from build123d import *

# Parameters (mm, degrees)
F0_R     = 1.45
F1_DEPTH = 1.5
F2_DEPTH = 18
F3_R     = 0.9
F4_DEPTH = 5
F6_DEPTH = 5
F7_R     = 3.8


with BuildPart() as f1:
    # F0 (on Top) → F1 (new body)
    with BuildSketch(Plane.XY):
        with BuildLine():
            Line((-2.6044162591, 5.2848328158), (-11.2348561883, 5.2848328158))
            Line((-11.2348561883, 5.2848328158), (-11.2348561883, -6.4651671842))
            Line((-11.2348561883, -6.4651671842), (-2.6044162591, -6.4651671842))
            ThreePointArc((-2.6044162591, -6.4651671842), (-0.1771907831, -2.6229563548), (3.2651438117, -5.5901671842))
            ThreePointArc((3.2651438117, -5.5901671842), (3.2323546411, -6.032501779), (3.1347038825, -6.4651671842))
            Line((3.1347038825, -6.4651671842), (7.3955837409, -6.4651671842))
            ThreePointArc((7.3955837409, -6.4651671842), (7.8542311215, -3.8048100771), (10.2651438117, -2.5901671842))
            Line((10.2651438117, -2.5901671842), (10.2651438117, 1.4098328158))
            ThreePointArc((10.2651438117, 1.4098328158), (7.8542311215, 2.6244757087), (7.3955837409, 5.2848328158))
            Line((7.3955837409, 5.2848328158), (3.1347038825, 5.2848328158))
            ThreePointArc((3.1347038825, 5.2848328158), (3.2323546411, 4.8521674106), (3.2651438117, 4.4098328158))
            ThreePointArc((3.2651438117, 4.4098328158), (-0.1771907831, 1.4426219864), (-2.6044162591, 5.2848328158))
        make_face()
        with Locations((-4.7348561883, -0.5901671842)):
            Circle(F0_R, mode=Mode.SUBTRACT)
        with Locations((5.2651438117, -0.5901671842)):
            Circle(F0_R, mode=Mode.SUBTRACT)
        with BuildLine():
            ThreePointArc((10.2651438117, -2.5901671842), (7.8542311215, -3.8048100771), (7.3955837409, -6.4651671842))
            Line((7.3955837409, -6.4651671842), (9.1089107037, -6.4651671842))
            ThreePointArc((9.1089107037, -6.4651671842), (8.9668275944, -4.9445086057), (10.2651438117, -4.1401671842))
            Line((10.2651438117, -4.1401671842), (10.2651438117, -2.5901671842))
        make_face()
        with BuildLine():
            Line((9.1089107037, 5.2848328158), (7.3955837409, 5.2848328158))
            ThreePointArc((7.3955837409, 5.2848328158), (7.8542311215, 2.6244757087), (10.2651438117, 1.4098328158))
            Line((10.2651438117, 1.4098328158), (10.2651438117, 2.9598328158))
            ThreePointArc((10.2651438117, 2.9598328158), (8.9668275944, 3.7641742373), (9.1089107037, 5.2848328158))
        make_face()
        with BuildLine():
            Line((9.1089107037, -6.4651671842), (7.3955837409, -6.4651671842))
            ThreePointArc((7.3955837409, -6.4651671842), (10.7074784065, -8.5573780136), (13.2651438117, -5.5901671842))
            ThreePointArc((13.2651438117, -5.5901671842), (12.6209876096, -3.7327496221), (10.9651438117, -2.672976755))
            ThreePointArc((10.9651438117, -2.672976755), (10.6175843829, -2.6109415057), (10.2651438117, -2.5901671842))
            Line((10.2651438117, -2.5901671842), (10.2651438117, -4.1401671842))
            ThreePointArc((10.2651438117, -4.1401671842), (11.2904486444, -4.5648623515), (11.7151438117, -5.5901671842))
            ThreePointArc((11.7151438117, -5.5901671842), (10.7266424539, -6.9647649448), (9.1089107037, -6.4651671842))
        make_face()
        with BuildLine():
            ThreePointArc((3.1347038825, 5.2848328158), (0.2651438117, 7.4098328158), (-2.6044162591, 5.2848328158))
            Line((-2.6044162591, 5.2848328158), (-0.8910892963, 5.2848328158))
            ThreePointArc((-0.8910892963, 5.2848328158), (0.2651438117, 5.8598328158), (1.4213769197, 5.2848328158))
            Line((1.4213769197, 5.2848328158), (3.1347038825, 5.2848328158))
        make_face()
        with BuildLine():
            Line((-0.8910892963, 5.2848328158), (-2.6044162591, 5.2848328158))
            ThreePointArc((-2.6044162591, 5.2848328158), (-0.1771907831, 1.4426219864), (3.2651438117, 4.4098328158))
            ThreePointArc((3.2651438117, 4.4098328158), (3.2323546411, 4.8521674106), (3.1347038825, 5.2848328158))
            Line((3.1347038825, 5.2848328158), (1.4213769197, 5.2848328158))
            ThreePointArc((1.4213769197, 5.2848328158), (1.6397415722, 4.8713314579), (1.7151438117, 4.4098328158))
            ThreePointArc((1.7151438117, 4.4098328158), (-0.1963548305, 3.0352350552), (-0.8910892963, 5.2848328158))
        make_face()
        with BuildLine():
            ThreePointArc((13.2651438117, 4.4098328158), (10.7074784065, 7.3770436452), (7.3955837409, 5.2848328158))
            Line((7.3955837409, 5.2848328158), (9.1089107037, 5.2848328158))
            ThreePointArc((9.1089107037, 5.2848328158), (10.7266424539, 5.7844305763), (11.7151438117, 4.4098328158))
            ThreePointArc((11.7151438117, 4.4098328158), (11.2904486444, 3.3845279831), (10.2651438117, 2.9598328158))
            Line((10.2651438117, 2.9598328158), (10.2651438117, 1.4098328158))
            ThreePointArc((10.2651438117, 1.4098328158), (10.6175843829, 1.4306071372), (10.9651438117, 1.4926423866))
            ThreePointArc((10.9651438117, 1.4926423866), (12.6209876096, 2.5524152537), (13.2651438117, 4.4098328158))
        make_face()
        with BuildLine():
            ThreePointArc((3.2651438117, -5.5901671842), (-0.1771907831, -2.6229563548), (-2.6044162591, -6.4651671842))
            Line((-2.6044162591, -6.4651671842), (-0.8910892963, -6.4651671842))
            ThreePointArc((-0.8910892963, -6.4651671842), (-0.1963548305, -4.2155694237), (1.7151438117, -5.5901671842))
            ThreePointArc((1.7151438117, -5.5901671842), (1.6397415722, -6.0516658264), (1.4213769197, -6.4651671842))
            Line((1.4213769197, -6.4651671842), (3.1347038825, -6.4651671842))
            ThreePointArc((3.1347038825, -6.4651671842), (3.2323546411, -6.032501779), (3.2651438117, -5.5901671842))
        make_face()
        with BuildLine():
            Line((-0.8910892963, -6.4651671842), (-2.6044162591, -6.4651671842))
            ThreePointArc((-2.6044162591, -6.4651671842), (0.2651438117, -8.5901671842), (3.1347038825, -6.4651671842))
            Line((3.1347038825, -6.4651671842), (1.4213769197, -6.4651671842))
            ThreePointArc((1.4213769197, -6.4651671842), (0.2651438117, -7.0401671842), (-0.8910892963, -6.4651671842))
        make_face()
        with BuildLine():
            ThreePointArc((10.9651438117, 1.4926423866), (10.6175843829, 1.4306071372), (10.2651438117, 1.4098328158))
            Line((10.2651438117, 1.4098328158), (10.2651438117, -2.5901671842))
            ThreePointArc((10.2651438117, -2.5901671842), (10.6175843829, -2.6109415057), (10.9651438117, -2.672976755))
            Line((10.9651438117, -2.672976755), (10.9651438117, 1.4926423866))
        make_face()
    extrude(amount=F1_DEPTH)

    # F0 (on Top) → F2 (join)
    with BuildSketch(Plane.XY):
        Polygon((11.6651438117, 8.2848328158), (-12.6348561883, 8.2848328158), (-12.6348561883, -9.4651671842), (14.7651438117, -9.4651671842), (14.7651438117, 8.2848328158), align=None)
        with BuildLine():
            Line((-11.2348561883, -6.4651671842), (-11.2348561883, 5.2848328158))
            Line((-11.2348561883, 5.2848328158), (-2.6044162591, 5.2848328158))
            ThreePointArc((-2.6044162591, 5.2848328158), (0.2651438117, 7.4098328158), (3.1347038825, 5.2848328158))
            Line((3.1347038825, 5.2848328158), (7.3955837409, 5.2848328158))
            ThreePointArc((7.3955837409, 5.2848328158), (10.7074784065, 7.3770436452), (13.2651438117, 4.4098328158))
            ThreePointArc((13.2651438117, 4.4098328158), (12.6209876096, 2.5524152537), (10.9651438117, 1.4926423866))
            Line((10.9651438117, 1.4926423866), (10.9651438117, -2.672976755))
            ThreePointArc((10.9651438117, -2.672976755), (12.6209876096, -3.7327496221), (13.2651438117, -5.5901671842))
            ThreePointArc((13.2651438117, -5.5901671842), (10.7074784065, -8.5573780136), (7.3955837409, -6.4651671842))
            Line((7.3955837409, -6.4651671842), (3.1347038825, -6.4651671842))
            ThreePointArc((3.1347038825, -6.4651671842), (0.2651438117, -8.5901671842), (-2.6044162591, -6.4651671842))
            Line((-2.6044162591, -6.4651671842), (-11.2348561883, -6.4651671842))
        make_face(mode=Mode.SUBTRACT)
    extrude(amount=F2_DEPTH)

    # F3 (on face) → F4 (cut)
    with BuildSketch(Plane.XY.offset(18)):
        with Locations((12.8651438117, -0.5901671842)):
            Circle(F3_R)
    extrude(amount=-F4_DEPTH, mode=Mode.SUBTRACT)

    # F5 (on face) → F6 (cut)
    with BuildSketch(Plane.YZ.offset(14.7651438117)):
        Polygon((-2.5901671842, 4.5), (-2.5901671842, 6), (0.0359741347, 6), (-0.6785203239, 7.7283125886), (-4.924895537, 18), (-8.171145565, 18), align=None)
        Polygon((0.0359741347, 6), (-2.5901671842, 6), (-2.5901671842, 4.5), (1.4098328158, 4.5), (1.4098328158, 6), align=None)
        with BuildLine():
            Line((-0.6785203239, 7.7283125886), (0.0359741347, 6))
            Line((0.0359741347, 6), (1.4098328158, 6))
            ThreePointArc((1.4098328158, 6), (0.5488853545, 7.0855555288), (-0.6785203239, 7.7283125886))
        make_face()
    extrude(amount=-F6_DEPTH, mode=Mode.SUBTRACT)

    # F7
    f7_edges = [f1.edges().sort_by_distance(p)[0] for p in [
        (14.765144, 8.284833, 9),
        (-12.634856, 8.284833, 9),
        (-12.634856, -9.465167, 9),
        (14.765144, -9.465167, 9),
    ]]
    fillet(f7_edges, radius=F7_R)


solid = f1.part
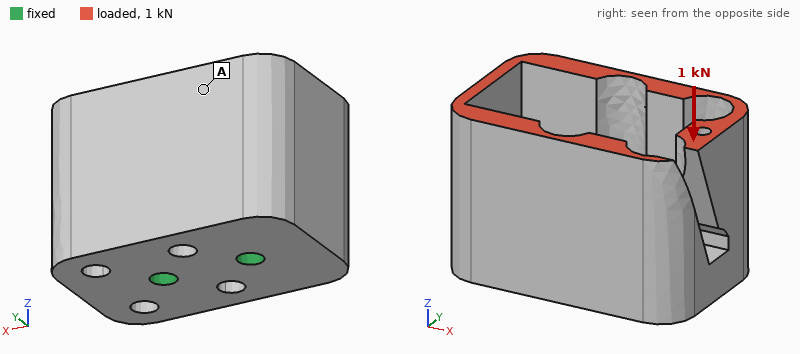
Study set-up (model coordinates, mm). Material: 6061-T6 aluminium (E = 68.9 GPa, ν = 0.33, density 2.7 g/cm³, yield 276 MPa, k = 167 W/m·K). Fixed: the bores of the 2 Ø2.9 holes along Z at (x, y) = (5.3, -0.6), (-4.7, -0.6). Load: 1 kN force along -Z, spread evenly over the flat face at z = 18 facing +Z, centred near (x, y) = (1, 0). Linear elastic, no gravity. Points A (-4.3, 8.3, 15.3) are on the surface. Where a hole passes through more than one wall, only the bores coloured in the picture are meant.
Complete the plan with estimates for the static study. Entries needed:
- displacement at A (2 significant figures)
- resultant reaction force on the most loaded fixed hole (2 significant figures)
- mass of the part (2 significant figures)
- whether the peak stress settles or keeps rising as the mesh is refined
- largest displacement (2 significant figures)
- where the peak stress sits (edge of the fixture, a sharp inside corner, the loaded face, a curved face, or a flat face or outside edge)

35 µm
520 N
8.7 g
keeps rising
45 µm
edge of the fixture
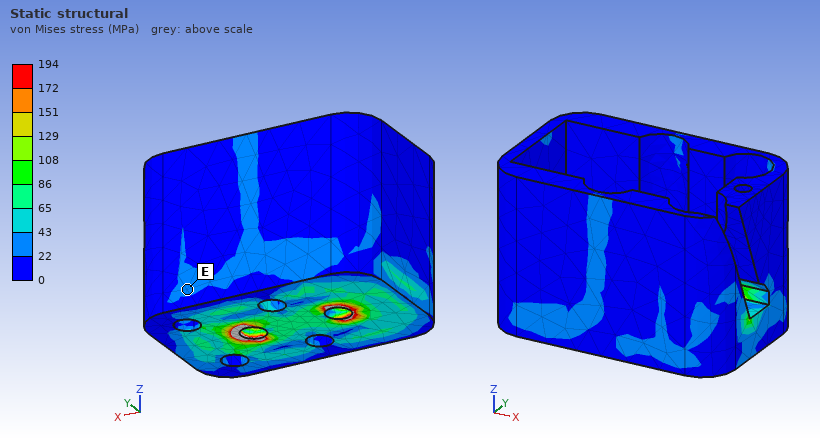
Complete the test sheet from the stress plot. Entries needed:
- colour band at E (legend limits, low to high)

22 to 43 MPa
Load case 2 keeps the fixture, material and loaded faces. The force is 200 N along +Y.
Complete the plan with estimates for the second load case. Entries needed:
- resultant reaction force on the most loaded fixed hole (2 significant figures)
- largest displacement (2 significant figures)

100 N
0.20 mm
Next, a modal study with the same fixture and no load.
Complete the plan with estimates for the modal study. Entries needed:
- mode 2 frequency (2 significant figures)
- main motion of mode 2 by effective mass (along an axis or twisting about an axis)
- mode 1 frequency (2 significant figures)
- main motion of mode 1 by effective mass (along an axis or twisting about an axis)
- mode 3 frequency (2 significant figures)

4900 Hz
along X
3100 Hz
along Y
6400 Hz
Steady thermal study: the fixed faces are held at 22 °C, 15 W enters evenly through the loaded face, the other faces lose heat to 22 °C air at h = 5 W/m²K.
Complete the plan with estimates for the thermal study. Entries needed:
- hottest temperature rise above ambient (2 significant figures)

25 K
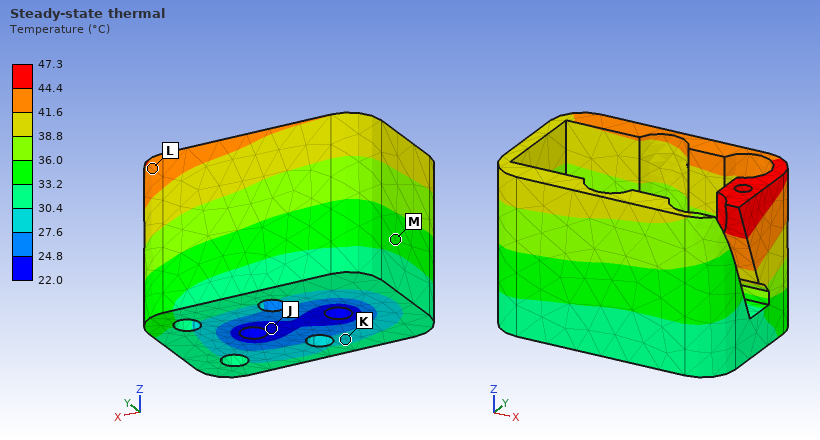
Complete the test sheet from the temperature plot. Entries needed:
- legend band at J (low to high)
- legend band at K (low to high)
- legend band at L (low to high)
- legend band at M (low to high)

22.0 to 24.8 °C
27.6 to 30.4 °C
41.6 to 44.4 °C
33.2 to 36.0 °C
